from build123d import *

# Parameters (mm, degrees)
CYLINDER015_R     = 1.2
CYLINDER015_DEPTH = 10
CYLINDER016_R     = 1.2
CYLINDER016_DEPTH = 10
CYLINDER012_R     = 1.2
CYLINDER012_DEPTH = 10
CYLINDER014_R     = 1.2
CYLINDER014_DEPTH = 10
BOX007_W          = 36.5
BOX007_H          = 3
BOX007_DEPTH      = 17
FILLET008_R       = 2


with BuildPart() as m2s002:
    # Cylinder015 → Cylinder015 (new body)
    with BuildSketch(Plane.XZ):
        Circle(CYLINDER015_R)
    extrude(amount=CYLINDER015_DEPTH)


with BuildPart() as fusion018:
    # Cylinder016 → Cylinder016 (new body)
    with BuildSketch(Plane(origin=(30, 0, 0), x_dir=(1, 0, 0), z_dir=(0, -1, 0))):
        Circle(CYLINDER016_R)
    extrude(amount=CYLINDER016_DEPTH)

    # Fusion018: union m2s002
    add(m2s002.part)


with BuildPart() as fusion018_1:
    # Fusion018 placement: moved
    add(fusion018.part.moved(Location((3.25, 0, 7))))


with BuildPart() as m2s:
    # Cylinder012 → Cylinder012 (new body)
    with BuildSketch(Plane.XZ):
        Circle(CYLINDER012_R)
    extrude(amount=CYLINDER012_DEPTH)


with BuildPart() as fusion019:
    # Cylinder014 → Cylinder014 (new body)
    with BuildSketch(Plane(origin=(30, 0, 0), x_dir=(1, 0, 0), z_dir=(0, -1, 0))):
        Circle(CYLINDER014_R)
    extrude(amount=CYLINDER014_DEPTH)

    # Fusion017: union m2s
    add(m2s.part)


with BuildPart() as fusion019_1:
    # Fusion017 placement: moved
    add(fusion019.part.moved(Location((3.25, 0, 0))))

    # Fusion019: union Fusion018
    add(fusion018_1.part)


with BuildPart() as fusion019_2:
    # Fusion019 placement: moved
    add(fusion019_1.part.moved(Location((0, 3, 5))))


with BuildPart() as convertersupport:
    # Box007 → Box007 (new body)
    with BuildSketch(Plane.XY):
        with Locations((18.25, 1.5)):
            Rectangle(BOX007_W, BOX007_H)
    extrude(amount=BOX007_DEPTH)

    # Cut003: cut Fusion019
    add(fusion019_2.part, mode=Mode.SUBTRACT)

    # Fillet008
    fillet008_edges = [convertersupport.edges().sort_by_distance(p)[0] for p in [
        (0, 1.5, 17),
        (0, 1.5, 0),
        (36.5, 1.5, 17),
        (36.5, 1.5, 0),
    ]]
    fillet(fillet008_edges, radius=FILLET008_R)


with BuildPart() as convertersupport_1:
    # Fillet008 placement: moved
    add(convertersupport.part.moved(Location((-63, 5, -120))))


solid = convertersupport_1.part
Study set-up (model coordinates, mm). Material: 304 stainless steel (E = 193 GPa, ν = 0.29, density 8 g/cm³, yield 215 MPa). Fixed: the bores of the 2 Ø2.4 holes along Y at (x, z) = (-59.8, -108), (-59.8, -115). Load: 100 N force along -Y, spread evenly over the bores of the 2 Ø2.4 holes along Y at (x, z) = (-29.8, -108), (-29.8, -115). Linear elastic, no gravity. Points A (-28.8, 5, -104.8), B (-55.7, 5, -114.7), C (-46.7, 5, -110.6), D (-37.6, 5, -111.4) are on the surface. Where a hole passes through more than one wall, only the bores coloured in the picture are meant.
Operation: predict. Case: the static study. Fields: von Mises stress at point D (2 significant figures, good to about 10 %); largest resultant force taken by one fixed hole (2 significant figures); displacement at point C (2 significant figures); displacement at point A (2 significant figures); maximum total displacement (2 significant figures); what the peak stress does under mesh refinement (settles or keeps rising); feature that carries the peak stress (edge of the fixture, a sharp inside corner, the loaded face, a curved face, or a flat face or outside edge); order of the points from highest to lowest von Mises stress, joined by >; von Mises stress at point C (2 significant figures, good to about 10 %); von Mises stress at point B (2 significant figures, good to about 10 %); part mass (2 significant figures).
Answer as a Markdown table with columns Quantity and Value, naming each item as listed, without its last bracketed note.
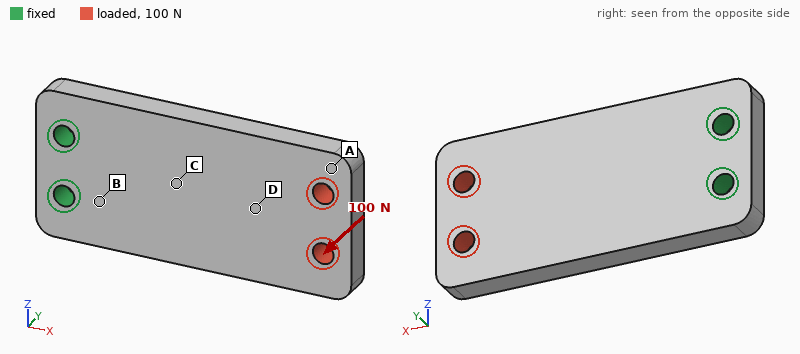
| Quantity | Value |
|---|---|
| von Mises stress at point D | 32 MPa |
| largest resultant force taken by one fixed hole | 50 N |
| displacement at point C | 0.029 mm |
| displacement at point A | 0.12 mm |
| maximum total displacement | 0.14 mm |
| what the peak stress does under mesh refinement | keeps rising |
| feature that carries the peak stress | edge of the fixture |
| order of the points from highest to lowest von Mises stress, joined by > | B > C > D > A |
| von Mises stress at point C | 63 MPa |
| von Mises stress at point B | 100 MPa |
| part mass | 14 g |
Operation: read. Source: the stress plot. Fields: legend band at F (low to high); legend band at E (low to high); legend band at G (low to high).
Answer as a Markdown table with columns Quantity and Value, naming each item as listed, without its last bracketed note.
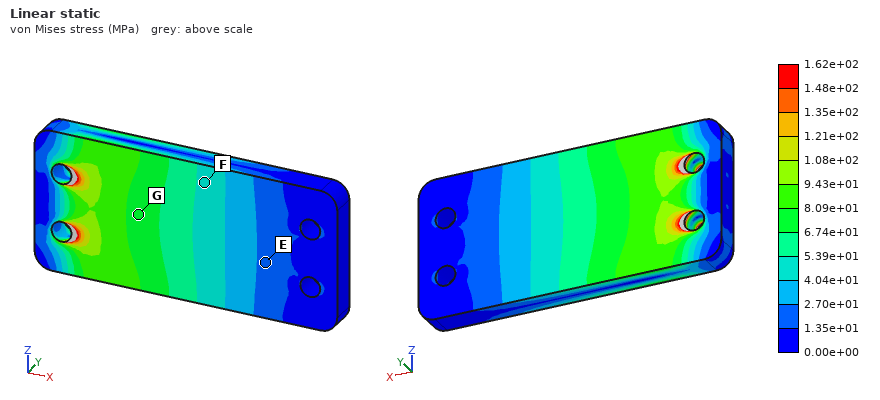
| Quantity | Value |
|---|---|
| legend band at F | 4.04e+01 to 5.39e+01 MPa |
| legend band at E | 1.35e+01 to 2.70e+01 MPa |
| legend band at G | 6.74e+01 to 8.09e+01 MPa |
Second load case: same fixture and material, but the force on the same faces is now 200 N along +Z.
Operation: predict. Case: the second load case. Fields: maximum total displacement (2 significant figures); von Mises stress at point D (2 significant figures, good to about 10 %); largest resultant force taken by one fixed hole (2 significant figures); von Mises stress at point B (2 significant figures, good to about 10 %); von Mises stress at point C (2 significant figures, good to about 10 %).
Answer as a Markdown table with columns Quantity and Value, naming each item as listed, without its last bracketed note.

| Quantity | Value |
|---|---|
| maximum total displacement | 15 µm |
| von Mises stress at point D | 10 MPa |
| largest resultant force taken by one fixed hole | 670 N |
| von Mises stress at point B | 29 MPa |
| von Mises stress at point C | 11 MPa |
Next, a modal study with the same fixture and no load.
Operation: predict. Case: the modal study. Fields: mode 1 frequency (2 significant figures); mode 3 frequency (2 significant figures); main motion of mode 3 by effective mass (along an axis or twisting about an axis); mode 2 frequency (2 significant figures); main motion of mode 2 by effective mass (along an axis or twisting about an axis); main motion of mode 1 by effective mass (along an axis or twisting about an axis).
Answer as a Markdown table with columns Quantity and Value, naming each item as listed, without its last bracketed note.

| Quantity | Value |
|---|---|
| mode 1 frequency | 2300 Hz |
| mode 3 frequency | 9000 Hz |
| main motion of mode 3 by effective mass | along Z |
| mode 2 frequency | 8500 Hz |
| main motion of mode 2 by effective mass | twisting about X |
| main motion of mode 1 by effective mass | along Y |
